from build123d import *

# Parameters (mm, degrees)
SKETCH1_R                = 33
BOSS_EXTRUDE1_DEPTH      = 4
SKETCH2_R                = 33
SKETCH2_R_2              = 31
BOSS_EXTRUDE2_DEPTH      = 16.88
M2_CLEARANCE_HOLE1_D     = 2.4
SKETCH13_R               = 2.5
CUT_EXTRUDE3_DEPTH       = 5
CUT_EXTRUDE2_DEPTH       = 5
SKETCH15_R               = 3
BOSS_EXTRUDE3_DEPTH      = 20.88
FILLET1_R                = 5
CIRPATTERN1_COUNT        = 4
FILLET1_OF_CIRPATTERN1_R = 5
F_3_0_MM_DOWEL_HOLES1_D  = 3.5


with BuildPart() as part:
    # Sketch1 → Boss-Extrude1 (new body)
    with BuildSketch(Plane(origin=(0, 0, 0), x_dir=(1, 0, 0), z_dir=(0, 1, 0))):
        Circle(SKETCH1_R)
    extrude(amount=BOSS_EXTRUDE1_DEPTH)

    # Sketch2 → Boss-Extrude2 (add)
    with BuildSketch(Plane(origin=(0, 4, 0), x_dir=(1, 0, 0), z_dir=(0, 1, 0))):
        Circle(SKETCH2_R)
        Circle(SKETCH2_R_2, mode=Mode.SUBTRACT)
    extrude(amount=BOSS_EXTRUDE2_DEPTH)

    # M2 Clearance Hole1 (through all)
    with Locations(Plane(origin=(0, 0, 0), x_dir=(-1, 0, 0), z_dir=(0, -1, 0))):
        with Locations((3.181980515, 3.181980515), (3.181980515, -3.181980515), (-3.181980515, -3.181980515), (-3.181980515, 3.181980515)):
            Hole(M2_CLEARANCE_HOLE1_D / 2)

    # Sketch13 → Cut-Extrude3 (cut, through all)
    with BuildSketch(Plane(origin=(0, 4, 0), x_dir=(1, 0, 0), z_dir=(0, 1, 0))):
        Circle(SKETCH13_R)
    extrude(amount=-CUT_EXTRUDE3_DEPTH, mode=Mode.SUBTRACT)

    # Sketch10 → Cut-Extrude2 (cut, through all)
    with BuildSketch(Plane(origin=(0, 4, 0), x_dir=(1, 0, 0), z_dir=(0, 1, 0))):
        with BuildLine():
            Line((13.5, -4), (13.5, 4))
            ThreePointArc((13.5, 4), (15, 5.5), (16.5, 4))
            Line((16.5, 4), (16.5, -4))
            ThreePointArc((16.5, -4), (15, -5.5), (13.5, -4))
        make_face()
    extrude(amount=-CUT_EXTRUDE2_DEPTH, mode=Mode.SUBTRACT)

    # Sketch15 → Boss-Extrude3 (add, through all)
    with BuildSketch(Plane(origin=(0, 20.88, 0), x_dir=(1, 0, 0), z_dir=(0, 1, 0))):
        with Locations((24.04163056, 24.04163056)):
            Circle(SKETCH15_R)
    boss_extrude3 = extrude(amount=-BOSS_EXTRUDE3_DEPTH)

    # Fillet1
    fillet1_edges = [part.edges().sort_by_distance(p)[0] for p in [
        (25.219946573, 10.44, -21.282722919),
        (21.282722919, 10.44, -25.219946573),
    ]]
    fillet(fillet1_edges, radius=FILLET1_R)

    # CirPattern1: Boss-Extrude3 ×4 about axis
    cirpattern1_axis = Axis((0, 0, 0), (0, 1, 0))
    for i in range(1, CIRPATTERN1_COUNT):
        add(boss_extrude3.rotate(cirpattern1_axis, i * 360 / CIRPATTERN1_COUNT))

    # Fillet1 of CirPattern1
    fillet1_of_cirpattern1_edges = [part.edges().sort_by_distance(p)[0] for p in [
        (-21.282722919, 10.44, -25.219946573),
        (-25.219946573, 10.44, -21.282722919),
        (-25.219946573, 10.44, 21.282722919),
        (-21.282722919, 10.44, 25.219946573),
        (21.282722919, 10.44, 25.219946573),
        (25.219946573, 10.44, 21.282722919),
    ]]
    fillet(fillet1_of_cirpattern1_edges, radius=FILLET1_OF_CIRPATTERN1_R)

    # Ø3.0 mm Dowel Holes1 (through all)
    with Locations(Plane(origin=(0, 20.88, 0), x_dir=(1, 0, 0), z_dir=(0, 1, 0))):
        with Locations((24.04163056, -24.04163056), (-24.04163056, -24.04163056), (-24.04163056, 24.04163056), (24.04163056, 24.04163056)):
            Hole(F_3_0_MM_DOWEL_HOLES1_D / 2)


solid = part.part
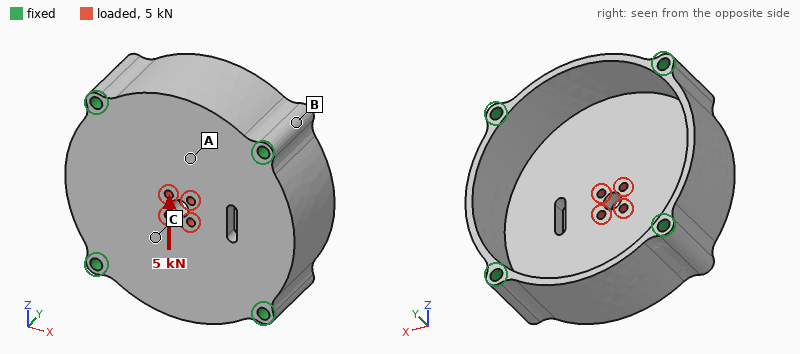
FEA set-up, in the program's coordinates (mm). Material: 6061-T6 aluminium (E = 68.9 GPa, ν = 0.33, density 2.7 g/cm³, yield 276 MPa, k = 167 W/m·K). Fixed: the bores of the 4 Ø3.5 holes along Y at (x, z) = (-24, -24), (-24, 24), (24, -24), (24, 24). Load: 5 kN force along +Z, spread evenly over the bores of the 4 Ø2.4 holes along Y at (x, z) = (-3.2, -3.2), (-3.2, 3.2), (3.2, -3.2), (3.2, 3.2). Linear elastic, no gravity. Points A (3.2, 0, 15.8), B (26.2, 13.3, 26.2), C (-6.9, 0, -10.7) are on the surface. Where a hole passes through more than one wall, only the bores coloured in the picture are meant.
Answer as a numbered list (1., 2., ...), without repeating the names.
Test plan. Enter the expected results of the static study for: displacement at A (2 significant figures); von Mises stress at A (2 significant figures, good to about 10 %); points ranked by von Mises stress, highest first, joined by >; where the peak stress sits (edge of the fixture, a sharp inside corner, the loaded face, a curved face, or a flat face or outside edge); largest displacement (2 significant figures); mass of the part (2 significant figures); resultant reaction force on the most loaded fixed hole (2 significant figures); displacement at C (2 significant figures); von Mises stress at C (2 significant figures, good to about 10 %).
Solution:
1. 11 µm
2. 14 MPa
3. C > A > B
4. the loaded face
5. 18 µm
6. 58 g
7. 1.4 kN
8. 10 µm
9. 25 MPa
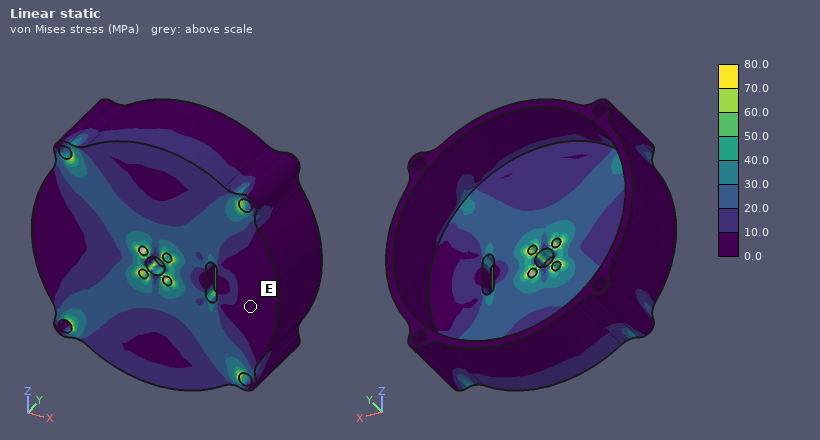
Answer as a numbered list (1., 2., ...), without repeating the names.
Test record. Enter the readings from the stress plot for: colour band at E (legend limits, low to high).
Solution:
1. 0.0 to 10.0 MPa
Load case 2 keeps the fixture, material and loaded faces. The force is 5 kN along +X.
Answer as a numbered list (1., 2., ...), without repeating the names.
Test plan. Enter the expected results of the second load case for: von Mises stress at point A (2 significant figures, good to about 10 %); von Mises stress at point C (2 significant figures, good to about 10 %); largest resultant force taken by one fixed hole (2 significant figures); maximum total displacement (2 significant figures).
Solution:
1. 13 MPa
2. 25 MPa
3. 1.3 kN
4. 19 µm
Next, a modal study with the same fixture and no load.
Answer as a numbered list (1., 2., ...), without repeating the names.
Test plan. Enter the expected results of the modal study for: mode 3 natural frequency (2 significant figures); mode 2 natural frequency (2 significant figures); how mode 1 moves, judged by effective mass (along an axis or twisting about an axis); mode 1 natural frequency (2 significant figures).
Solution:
1. 14 kHz
2. 14 kHz
3. along Y
4. 7000 Hz
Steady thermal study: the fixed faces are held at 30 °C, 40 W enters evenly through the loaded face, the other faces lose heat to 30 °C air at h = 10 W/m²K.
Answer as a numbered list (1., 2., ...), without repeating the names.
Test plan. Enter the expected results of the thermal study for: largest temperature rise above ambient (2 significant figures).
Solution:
1. 26 K
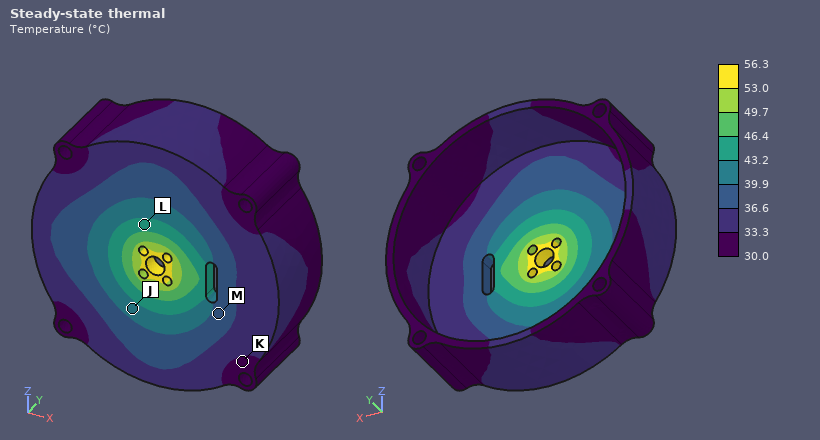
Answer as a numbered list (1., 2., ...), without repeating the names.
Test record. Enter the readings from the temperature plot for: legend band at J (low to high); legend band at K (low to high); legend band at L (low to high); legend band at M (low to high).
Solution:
1. 39.9 to 43.2 °C
2. 30.0 to 33.3 °C
3. 43.2 to 46.4 °C
4. 36.6 to 39.9 °C
